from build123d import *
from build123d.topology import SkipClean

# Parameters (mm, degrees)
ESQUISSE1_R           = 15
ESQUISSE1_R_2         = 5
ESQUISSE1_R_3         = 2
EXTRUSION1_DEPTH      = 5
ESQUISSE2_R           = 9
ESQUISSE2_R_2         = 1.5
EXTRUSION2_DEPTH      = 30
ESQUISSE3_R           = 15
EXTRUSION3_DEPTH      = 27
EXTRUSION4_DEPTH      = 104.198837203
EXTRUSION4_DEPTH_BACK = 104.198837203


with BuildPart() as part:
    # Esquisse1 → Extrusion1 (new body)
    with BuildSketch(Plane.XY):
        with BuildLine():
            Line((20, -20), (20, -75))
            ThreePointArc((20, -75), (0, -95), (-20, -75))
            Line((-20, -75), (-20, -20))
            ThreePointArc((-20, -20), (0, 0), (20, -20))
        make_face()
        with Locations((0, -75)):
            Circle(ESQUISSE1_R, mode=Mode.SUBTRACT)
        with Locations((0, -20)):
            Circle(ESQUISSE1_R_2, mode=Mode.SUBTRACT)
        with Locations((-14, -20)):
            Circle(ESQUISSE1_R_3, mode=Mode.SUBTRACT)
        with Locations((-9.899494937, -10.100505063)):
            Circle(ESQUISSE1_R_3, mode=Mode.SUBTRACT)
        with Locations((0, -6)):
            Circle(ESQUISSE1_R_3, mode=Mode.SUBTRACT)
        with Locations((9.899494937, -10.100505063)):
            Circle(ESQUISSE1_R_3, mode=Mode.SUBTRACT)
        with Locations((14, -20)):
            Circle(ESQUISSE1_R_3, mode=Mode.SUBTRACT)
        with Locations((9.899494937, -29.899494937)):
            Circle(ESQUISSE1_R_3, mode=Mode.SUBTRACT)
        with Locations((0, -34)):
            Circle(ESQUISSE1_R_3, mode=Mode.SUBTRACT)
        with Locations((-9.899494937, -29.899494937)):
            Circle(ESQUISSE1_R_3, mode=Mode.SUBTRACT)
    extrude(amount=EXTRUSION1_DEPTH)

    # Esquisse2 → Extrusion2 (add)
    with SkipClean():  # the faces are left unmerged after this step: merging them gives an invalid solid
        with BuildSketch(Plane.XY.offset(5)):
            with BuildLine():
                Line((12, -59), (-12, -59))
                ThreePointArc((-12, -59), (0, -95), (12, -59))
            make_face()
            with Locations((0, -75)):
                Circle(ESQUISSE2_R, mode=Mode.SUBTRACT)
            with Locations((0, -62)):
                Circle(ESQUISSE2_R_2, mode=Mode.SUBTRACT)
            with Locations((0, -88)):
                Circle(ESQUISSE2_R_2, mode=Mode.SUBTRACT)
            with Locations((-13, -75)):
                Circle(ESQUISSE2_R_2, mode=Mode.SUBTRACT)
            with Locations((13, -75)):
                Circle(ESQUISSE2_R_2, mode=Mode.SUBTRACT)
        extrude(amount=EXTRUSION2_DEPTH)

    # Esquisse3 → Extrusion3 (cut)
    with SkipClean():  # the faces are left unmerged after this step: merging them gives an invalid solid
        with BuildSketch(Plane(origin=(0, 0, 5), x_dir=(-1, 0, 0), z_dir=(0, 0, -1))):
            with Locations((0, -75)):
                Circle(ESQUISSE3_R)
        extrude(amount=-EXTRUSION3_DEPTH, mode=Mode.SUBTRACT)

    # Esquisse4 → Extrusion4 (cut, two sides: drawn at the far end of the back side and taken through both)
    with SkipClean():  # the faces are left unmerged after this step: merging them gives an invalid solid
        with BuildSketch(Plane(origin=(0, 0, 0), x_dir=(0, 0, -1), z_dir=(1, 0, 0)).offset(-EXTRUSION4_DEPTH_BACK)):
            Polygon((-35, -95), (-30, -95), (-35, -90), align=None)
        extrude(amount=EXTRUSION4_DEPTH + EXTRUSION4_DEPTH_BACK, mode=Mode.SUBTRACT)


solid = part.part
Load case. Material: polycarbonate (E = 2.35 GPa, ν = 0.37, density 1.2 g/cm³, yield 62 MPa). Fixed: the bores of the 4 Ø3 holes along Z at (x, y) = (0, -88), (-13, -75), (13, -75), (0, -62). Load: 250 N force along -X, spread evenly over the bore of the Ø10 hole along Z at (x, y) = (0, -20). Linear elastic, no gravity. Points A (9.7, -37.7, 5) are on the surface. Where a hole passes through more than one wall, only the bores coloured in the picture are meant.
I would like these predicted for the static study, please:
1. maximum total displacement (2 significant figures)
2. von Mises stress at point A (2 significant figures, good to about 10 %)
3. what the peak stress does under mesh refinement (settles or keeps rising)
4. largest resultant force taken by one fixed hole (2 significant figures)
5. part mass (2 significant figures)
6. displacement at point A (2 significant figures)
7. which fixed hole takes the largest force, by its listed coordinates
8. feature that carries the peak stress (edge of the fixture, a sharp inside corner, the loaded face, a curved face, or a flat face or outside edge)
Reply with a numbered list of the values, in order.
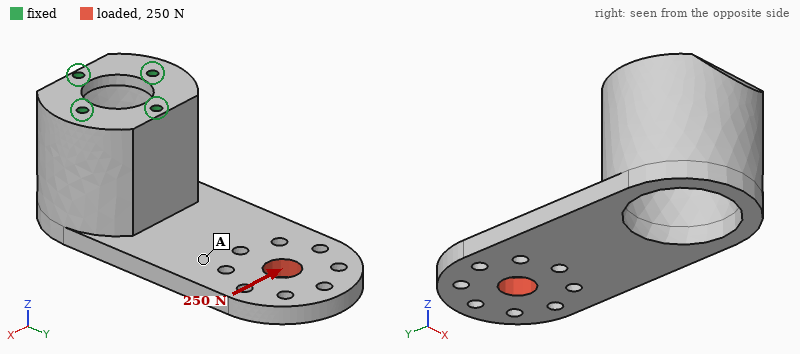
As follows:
1. 1.2 mm
2. 3.5 MPa
3. keeps rising
4. 390 N
5. 34 g
6. 0.60 mm
7. (0, -62)
8. edge of the fixture
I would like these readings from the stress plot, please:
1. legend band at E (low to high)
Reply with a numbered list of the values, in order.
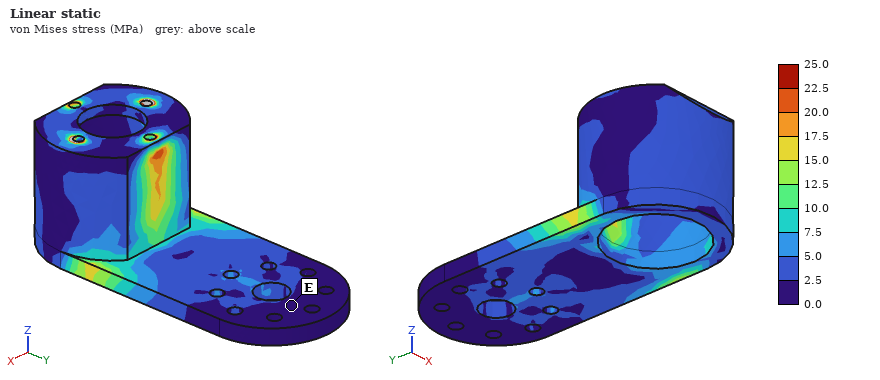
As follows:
1. 0.0 to 2.5 MPa
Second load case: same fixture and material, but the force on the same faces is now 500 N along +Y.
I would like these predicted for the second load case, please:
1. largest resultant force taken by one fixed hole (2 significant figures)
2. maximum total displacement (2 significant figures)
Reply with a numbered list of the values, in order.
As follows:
1. 510 N
2. 1.2 mm
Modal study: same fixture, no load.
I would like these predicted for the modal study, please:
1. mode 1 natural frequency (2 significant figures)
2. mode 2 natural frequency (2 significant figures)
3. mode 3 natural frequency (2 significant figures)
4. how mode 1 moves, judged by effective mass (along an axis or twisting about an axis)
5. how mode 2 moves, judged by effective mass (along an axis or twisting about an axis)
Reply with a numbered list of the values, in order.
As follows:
1. 300 Hz
2. 870 Hz
3. 1000 Hz
4. along Z
5. along X
